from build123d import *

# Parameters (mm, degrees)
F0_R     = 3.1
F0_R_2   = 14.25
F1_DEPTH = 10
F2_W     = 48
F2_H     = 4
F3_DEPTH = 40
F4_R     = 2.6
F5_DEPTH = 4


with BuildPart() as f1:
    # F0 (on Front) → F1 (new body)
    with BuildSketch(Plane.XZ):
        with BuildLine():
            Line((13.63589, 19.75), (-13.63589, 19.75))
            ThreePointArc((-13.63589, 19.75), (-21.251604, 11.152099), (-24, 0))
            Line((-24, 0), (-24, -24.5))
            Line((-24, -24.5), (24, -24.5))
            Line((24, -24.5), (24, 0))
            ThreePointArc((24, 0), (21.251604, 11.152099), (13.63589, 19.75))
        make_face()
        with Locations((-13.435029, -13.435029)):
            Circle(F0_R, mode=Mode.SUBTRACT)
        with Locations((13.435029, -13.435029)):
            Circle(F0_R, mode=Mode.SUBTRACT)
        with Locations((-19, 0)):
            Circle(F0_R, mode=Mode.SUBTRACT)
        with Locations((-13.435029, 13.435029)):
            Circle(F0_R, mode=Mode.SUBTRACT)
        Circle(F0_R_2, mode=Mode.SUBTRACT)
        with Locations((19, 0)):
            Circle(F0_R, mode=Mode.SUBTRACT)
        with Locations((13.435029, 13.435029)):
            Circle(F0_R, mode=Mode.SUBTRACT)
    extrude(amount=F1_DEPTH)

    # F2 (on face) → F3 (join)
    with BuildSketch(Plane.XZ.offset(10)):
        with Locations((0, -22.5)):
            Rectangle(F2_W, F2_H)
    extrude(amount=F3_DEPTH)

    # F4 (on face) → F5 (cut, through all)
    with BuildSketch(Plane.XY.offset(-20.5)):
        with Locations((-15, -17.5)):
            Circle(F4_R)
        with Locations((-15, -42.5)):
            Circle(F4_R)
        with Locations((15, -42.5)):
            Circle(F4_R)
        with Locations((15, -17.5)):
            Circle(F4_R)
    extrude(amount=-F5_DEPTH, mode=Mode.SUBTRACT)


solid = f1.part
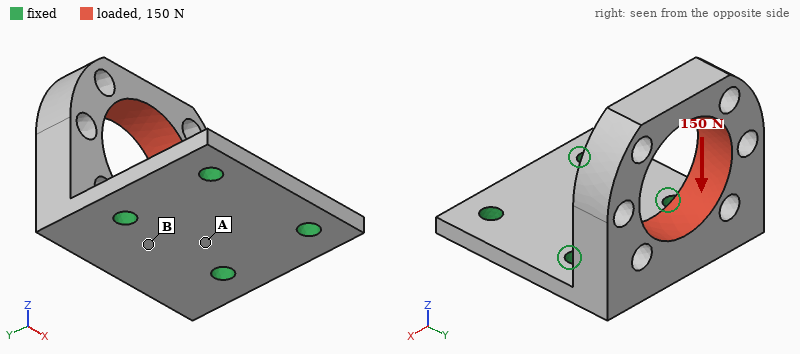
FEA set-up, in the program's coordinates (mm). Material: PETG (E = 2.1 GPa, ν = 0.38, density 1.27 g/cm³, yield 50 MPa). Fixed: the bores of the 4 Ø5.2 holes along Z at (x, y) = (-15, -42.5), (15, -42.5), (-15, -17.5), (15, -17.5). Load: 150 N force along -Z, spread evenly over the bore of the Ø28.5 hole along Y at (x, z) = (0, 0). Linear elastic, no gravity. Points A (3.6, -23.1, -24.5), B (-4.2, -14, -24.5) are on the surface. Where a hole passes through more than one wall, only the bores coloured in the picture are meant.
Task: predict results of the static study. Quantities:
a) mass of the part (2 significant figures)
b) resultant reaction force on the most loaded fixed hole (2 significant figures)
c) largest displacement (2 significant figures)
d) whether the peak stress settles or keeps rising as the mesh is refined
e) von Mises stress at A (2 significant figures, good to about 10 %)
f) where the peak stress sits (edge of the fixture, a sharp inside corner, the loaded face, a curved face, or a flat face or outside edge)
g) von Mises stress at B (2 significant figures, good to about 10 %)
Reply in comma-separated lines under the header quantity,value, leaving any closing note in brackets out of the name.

quantity,value
mass of the part,24 g
resultant reaction force on the most loaded fixed hole,81 N
largest displacement,0.80 mm
whether the peak stress settles or keeps rising as the mesh is refined,keeps rising
von Mises stress at A,2.0 MPa
where the peak stress sits,edge of the fixture
von Mises stress at B,5.2 MPa
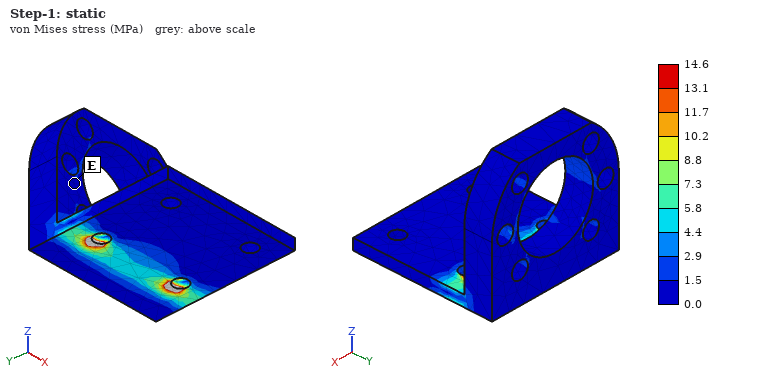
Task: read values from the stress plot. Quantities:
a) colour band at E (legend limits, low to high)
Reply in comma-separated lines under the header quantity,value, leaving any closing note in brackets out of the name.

quantity,value
colour band at E,0.0 to 1.5 MPa
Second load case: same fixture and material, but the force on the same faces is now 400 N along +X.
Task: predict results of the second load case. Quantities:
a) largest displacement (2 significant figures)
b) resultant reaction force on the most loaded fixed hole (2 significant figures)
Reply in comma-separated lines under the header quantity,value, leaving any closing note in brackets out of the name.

quantity,value
largest displacement,0.93 mm
resultant reaction force on the most loaded fixed hole,360 N
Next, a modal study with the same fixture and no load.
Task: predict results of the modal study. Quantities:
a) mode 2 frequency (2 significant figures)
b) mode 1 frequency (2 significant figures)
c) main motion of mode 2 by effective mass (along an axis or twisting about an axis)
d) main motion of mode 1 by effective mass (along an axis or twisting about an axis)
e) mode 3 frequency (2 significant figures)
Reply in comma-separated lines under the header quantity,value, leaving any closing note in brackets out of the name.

quantity,value
mode 2 frequency,1100 Hz
mode 1 frequency,420 Hz
main motion of mode 2 by effective mass,along X
main motion of mode 1 by effective mass,along Y
mode 3 frequency,1700 Hz
